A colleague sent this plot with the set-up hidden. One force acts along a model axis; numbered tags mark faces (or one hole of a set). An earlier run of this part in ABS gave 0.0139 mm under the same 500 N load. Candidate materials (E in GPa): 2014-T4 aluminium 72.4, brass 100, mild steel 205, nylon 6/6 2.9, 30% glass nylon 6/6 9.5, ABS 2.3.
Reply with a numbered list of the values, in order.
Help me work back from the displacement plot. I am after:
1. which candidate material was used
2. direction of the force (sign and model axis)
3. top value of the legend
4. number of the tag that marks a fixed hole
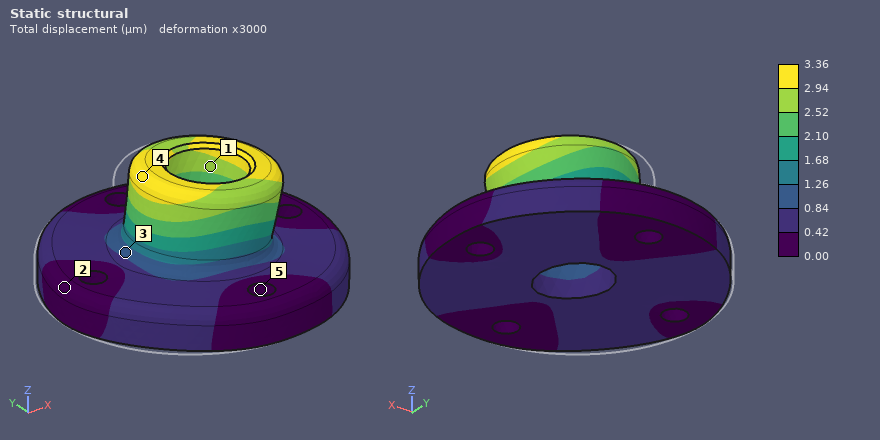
1. 30% glass nylon 6/6
2. +X
3. 3.36 µm
4. 5
